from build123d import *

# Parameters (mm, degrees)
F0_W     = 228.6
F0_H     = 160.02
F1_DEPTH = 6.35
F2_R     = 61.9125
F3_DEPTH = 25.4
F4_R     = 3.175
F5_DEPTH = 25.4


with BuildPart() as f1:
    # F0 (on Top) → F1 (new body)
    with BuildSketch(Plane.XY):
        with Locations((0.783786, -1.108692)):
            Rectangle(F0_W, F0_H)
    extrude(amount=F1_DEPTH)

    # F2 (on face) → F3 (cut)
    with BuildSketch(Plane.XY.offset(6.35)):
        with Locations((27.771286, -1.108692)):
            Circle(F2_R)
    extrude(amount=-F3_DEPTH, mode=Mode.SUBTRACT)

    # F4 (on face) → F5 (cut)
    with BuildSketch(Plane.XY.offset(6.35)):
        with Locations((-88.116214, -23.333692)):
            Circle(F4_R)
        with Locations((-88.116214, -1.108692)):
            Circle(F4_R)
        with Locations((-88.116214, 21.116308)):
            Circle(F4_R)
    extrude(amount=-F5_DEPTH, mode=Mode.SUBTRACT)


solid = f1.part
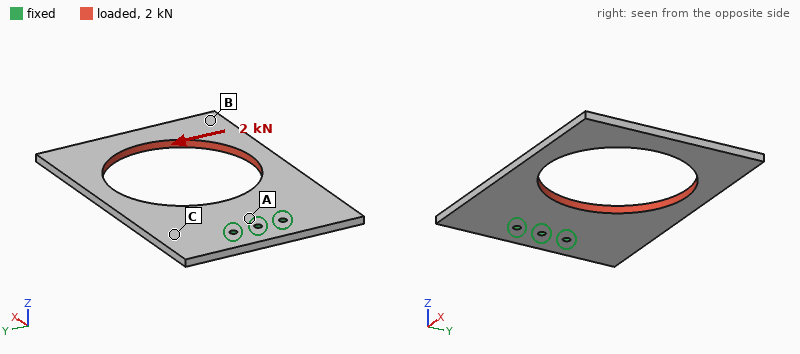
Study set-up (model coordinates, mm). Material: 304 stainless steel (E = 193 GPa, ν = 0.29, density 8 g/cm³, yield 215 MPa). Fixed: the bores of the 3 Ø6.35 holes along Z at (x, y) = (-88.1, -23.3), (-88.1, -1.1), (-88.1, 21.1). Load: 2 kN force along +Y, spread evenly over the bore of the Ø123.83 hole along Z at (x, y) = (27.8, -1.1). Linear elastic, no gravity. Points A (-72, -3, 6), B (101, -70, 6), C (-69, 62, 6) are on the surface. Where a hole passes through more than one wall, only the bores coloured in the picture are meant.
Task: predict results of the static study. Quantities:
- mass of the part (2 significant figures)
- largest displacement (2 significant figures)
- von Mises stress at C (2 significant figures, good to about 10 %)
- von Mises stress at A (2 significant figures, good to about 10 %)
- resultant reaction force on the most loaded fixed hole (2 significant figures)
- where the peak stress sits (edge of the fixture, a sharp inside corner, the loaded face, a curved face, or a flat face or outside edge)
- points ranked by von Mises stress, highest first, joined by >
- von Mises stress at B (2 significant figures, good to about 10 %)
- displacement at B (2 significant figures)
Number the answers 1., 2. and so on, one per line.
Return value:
1. 1.2 kg
2. 88 µm
3. 6.5 MPa
4. 22 MPa
5. 4.7 kN
6. edge of the fixture
7. A > C > B
8. 3.7 MPa
9. 84 µm
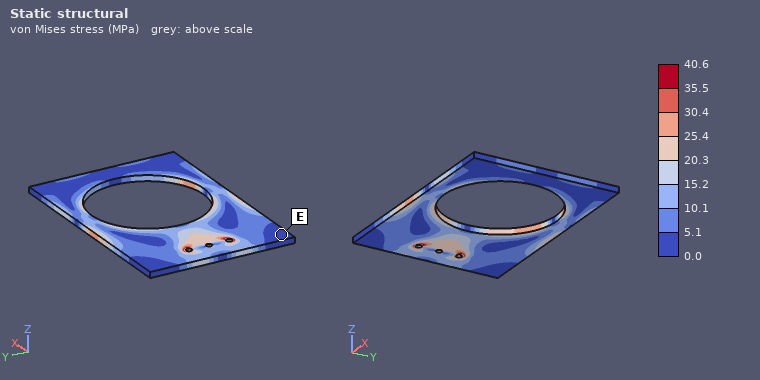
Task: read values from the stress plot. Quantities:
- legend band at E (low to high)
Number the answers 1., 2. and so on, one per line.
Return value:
1. 0.0 to 5.1 MPa
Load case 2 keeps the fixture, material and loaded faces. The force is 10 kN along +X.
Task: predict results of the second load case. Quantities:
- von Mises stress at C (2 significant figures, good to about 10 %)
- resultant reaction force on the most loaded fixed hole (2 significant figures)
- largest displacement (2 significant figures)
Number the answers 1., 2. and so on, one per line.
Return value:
1. 16 MPa
2. 4.9 kN
3. 58 µm
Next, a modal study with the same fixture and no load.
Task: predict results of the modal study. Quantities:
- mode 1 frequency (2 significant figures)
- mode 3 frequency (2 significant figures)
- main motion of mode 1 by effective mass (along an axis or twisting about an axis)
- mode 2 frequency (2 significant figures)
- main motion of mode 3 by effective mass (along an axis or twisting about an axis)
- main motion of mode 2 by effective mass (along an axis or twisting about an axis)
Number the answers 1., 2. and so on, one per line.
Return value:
1. 110 Hz
2. 620 Hz
3. along Z
4. 260 Hz
5. along Z
6. twisting about X
